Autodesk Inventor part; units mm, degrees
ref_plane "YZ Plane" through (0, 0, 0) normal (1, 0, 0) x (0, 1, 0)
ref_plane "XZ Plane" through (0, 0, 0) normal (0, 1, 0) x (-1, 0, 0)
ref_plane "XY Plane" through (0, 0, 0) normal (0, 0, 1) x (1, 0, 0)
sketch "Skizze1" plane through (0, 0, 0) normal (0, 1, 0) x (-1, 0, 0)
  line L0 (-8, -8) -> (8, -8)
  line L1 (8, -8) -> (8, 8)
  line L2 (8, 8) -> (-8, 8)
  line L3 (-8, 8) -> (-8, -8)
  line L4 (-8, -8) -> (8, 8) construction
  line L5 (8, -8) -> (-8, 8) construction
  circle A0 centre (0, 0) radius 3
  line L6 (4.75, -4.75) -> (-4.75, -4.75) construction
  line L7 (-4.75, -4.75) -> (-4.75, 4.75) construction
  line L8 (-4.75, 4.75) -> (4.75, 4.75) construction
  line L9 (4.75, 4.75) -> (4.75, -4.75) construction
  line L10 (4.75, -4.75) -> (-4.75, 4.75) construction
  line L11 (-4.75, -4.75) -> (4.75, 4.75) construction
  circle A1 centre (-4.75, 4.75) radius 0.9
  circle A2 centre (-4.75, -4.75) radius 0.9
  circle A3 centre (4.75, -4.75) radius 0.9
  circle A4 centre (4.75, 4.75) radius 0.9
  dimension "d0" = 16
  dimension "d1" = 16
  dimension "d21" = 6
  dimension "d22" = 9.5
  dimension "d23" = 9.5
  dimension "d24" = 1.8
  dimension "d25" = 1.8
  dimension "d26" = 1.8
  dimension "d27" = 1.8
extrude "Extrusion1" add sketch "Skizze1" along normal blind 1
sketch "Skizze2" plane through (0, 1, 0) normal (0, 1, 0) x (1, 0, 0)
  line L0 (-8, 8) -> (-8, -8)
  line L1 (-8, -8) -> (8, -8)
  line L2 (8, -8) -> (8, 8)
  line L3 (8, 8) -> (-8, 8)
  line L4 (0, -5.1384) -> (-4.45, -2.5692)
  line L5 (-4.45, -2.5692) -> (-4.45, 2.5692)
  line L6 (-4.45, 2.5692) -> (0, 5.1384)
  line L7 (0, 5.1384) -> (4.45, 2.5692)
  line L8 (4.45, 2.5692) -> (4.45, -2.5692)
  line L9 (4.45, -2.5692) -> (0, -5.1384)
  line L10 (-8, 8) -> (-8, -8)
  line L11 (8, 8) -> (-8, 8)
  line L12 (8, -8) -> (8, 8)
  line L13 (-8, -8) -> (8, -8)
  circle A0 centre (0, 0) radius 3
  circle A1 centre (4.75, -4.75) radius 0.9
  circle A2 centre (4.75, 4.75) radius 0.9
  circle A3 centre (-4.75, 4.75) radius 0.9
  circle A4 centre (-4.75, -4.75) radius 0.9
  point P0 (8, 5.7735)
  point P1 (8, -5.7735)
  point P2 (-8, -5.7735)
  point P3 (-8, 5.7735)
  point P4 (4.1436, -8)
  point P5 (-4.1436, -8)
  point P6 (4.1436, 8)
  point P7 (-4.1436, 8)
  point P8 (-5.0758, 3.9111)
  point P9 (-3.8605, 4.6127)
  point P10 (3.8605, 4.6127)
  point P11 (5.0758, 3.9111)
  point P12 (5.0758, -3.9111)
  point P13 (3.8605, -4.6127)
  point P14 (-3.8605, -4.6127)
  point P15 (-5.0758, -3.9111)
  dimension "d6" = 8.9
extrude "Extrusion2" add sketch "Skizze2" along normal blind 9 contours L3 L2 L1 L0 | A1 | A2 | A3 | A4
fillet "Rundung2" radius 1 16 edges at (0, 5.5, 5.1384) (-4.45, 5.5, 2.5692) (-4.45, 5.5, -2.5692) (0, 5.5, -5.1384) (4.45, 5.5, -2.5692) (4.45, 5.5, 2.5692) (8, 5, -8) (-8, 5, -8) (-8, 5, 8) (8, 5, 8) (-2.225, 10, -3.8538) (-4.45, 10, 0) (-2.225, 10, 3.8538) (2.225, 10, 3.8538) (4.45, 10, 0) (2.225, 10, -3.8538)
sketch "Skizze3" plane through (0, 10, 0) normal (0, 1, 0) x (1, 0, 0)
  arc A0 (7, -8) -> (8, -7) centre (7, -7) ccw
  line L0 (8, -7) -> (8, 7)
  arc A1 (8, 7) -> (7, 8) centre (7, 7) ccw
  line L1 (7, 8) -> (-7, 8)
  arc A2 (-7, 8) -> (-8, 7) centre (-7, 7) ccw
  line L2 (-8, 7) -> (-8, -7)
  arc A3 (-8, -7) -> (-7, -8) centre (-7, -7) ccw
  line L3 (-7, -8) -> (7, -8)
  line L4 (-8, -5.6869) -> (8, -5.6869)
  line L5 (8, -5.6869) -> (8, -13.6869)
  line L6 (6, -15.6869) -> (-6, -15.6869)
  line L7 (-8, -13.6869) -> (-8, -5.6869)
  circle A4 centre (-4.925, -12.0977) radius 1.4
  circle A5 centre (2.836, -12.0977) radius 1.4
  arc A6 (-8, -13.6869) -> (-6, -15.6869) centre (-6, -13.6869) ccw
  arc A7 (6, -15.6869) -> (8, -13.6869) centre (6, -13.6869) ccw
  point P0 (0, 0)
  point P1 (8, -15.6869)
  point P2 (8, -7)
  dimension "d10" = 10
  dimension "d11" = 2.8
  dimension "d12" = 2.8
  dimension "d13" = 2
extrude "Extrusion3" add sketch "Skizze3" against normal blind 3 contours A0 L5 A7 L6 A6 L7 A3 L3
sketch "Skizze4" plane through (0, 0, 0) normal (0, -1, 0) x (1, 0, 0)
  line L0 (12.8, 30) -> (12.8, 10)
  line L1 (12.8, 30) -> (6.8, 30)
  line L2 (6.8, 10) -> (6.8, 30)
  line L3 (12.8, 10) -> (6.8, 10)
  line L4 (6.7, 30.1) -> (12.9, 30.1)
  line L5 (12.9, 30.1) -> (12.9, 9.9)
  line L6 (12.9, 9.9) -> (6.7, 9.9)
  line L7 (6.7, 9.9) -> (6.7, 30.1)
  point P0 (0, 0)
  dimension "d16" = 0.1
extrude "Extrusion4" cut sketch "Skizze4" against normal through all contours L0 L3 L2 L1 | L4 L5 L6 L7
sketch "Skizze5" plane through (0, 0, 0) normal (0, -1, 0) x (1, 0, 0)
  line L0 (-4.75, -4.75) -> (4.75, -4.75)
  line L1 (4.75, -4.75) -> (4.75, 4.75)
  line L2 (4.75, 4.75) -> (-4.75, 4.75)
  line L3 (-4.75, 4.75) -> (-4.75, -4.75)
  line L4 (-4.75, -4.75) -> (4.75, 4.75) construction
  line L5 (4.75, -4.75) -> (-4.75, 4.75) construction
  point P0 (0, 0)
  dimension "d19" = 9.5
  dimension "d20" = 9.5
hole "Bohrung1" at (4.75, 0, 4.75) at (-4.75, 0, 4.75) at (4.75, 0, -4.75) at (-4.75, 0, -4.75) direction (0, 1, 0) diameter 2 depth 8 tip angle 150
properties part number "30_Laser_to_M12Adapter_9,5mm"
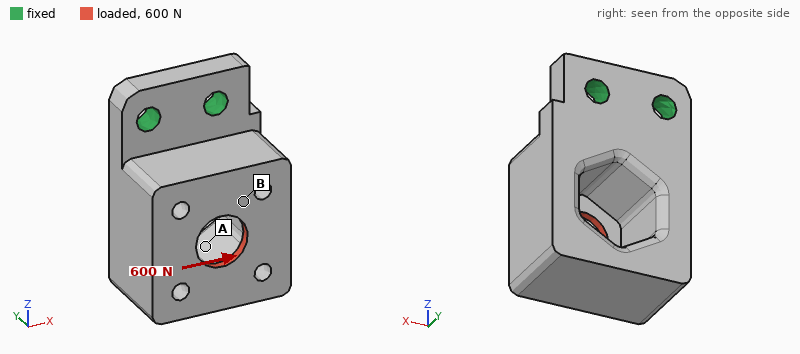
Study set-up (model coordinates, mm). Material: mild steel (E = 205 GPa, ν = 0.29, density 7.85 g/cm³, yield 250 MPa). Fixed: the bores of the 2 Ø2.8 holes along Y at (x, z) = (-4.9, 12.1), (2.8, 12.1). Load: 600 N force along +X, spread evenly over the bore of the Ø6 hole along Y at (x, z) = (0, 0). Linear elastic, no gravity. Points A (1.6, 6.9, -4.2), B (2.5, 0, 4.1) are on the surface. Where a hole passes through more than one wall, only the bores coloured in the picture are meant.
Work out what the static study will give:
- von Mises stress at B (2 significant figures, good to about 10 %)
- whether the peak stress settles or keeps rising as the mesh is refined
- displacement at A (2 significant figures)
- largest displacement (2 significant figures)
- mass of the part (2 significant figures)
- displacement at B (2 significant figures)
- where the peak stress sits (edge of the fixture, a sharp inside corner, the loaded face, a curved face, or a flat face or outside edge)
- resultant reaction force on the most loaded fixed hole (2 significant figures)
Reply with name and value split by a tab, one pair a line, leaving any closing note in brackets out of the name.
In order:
von Mises stress at B	41 MPa
whether the peak stress settles or keeps rising as the mesh is refined	keeps rising
displacement at A	6.9 µm
largest displacement	15 µm
mass of the part	17 g
displacement at B	8.9 µm
where the peak stress sits	edge of the fixture
resultant reaction force on the most loaded fixed hole	900 N
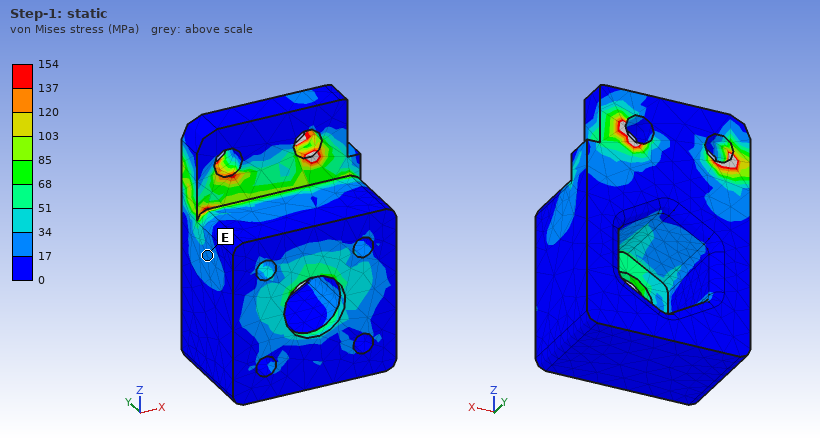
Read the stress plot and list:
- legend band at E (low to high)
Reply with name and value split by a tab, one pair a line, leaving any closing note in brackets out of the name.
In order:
legend band at E	17 to 34 MPa
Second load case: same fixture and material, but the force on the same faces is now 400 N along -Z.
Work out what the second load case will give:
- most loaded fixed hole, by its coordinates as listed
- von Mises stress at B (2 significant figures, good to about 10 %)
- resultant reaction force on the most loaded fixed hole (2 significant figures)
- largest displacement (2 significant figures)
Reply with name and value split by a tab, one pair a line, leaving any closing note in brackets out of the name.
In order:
most loaded fixed hole, by its coordinates as listed	(2.8, 12.1)
von Mises stress at B	27 MPa
resultant reaction force on the most loaded fixed hole	240 N
largest displacement	45 µm
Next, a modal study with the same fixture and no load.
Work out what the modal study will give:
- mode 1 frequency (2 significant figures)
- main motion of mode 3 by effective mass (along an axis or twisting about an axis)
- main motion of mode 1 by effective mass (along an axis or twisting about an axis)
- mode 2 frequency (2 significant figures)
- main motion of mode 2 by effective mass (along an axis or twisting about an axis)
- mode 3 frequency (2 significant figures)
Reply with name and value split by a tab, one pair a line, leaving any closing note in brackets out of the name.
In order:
mode 1 frequency	4300 Hz
main motion of mode 3 by effective mass	twisting about Z
main motion of mode 1 by effective mass	along Y
mode 2 frequency	12 kHz
main motion of mode 2 by effective mass	along X
mode 3 frequency	15 kHz
